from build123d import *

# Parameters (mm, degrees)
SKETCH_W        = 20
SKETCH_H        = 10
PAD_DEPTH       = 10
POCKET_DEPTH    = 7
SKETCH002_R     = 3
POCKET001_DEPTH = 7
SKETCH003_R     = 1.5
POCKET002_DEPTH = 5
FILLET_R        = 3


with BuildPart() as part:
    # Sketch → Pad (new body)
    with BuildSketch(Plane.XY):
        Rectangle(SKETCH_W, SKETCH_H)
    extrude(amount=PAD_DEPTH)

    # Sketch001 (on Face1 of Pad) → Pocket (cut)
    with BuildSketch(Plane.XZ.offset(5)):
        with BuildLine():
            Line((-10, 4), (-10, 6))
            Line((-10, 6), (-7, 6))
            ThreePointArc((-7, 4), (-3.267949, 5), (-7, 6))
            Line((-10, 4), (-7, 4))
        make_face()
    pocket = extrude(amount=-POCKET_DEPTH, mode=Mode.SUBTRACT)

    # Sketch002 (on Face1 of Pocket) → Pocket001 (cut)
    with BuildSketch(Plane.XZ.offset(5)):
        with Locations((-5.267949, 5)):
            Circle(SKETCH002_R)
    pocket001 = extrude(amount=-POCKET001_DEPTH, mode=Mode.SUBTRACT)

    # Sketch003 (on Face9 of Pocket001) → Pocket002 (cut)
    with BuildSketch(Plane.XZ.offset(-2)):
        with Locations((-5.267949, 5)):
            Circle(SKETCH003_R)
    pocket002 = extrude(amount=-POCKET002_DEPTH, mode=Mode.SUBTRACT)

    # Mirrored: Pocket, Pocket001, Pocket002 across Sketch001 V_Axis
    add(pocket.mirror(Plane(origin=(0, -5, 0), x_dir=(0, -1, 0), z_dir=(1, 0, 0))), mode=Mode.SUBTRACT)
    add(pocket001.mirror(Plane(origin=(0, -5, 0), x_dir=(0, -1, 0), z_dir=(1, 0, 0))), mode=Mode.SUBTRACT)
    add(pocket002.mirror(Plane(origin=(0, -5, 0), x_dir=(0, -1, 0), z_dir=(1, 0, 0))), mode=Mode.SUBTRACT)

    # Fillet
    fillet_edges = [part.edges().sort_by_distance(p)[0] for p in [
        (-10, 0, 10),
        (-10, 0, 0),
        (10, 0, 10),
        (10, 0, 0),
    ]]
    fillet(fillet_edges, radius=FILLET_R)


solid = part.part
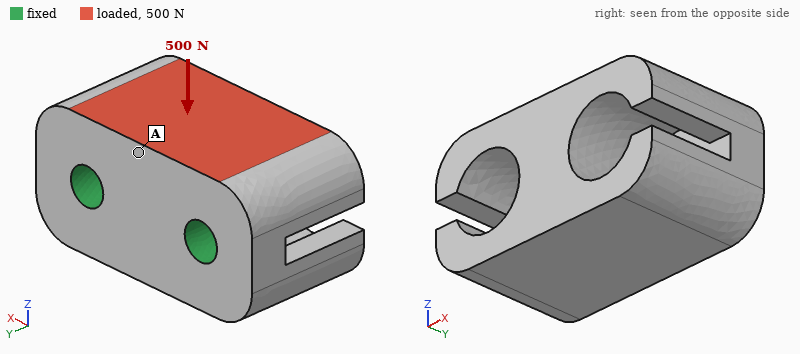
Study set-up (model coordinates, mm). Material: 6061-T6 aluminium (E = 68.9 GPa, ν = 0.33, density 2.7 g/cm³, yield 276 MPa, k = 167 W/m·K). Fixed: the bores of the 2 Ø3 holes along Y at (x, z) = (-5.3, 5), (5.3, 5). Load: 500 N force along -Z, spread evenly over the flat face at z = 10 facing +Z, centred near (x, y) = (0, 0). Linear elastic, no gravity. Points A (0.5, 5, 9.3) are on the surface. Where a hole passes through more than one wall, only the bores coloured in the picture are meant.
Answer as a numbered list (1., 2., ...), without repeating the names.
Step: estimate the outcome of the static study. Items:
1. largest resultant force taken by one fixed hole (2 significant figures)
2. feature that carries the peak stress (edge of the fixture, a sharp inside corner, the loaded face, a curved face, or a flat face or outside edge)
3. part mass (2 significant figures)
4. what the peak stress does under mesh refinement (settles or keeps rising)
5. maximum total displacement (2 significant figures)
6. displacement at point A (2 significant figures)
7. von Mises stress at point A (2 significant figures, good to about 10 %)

1. 250 N
2. edge of the fixture
3. 3.9 g
4. keeps rising
5. 8.6 µm
6. 2.6 µm
7. 8.7 MPa
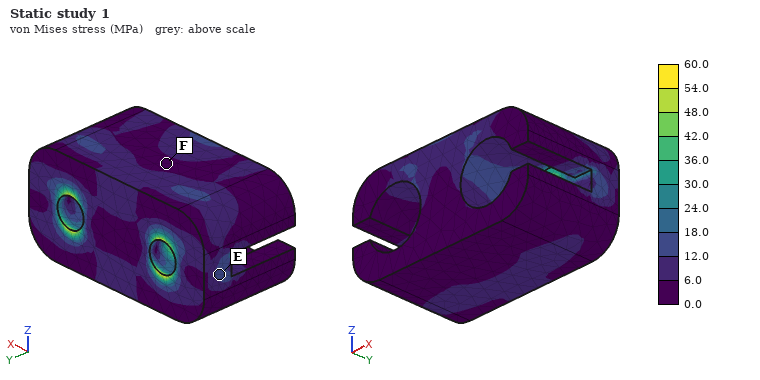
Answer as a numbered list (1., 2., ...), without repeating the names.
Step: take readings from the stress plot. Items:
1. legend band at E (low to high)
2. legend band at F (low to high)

1. 12.0 to 18.0 MPa
2. 0.0 to 6.0 MPa
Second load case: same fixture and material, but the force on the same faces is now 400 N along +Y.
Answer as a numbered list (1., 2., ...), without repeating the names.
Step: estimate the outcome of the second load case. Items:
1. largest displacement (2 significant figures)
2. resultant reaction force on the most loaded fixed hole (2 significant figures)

1. 7.9 µm
2. 210 N
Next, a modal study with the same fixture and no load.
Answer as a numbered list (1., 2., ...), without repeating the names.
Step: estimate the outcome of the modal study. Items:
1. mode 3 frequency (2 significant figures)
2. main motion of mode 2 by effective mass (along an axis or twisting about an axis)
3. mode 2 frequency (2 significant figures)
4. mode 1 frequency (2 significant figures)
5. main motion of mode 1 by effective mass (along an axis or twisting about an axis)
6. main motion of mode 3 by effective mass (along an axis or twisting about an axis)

1. 45 kHz
2. along X
3. 40 kHz
4. 26 kHz
5. along Z
6. twisting about Y
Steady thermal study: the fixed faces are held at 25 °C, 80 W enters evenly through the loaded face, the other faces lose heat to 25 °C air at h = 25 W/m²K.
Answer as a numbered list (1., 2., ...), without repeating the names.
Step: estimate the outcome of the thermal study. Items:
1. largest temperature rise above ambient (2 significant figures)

1. 41 K
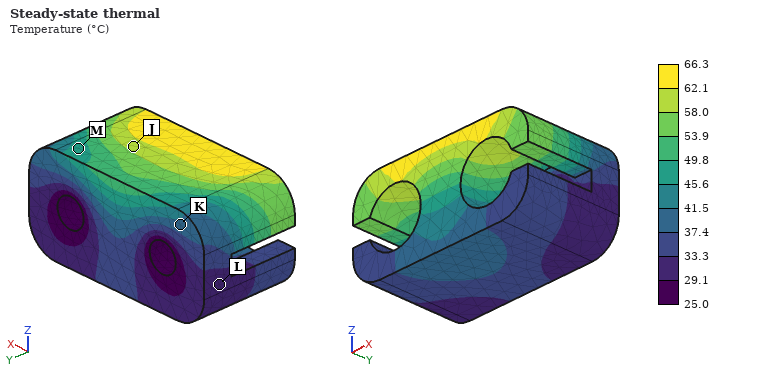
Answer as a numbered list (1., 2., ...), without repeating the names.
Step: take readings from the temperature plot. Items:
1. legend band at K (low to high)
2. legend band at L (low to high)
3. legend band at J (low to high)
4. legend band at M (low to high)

1. 37.4 to 41.5 °C
2. 29.1 to 33.3 °C
3. 58.0 to 62.1 °C
4. 45.6 to 49.8 °C
